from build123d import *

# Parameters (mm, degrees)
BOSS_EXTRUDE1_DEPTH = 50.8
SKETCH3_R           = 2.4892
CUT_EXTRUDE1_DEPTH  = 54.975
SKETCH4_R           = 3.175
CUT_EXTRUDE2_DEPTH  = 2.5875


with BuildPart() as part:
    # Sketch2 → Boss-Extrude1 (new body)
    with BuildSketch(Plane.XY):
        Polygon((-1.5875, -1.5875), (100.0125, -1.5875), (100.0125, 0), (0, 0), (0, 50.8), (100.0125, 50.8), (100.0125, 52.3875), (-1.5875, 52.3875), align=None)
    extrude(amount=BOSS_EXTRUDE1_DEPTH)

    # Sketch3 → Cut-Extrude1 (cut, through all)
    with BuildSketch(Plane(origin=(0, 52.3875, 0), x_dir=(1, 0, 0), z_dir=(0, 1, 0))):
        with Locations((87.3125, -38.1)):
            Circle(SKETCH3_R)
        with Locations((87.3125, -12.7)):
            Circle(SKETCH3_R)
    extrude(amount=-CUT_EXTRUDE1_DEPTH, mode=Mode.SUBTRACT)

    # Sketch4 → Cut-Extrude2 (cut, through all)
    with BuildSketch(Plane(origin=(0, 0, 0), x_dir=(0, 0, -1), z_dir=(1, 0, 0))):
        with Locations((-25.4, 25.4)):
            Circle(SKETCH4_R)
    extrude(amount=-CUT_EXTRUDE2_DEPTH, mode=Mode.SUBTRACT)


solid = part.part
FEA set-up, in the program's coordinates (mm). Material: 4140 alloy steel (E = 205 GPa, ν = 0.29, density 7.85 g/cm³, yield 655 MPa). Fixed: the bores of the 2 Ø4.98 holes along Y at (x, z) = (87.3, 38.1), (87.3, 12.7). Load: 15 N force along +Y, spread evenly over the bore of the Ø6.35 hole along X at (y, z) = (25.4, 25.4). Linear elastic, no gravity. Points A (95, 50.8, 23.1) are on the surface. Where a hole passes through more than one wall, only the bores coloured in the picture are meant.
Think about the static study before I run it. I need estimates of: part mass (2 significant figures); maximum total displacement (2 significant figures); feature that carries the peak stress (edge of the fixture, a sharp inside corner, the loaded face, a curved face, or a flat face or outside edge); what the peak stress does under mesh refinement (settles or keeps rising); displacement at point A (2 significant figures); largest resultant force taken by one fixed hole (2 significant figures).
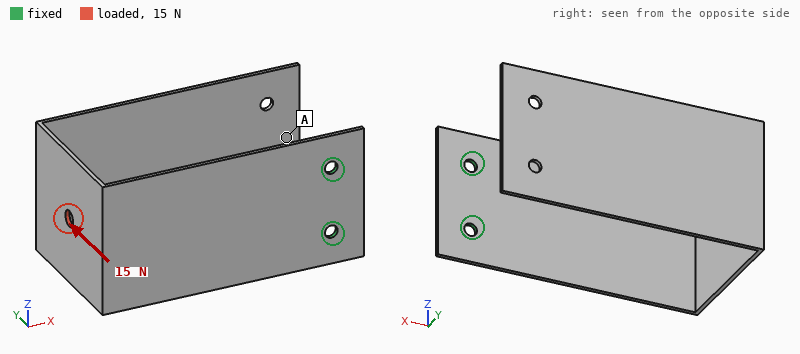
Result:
160 g
1.3 mm
edge of the fixture
keeps rising
1.0 mm
7.5 N
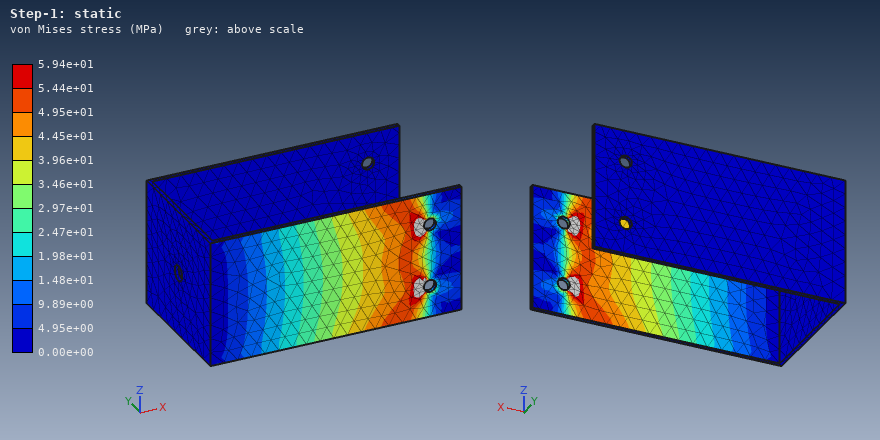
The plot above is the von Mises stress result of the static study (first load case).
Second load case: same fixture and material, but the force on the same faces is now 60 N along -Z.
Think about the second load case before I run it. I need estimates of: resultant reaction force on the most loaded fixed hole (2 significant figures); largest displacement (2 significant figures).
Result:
190 N
1.4 mm
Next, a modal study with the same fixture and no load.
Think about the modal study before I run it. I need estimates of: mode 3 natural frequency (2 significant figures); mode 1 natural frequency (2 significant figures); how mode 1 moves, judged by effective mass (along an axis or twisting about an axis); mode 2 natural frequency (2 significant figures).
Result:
75 Hz
49 Hz
along X
74 Hz
